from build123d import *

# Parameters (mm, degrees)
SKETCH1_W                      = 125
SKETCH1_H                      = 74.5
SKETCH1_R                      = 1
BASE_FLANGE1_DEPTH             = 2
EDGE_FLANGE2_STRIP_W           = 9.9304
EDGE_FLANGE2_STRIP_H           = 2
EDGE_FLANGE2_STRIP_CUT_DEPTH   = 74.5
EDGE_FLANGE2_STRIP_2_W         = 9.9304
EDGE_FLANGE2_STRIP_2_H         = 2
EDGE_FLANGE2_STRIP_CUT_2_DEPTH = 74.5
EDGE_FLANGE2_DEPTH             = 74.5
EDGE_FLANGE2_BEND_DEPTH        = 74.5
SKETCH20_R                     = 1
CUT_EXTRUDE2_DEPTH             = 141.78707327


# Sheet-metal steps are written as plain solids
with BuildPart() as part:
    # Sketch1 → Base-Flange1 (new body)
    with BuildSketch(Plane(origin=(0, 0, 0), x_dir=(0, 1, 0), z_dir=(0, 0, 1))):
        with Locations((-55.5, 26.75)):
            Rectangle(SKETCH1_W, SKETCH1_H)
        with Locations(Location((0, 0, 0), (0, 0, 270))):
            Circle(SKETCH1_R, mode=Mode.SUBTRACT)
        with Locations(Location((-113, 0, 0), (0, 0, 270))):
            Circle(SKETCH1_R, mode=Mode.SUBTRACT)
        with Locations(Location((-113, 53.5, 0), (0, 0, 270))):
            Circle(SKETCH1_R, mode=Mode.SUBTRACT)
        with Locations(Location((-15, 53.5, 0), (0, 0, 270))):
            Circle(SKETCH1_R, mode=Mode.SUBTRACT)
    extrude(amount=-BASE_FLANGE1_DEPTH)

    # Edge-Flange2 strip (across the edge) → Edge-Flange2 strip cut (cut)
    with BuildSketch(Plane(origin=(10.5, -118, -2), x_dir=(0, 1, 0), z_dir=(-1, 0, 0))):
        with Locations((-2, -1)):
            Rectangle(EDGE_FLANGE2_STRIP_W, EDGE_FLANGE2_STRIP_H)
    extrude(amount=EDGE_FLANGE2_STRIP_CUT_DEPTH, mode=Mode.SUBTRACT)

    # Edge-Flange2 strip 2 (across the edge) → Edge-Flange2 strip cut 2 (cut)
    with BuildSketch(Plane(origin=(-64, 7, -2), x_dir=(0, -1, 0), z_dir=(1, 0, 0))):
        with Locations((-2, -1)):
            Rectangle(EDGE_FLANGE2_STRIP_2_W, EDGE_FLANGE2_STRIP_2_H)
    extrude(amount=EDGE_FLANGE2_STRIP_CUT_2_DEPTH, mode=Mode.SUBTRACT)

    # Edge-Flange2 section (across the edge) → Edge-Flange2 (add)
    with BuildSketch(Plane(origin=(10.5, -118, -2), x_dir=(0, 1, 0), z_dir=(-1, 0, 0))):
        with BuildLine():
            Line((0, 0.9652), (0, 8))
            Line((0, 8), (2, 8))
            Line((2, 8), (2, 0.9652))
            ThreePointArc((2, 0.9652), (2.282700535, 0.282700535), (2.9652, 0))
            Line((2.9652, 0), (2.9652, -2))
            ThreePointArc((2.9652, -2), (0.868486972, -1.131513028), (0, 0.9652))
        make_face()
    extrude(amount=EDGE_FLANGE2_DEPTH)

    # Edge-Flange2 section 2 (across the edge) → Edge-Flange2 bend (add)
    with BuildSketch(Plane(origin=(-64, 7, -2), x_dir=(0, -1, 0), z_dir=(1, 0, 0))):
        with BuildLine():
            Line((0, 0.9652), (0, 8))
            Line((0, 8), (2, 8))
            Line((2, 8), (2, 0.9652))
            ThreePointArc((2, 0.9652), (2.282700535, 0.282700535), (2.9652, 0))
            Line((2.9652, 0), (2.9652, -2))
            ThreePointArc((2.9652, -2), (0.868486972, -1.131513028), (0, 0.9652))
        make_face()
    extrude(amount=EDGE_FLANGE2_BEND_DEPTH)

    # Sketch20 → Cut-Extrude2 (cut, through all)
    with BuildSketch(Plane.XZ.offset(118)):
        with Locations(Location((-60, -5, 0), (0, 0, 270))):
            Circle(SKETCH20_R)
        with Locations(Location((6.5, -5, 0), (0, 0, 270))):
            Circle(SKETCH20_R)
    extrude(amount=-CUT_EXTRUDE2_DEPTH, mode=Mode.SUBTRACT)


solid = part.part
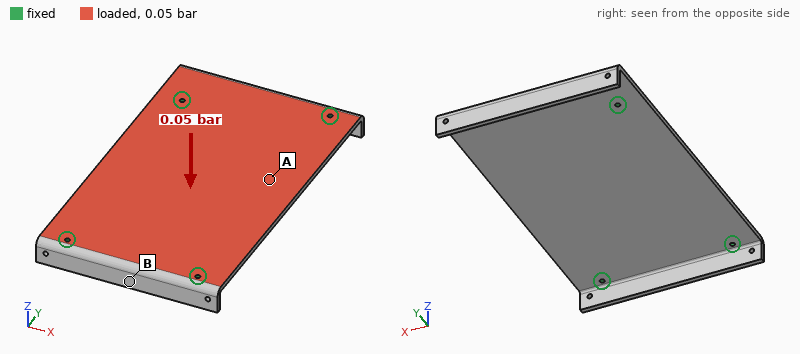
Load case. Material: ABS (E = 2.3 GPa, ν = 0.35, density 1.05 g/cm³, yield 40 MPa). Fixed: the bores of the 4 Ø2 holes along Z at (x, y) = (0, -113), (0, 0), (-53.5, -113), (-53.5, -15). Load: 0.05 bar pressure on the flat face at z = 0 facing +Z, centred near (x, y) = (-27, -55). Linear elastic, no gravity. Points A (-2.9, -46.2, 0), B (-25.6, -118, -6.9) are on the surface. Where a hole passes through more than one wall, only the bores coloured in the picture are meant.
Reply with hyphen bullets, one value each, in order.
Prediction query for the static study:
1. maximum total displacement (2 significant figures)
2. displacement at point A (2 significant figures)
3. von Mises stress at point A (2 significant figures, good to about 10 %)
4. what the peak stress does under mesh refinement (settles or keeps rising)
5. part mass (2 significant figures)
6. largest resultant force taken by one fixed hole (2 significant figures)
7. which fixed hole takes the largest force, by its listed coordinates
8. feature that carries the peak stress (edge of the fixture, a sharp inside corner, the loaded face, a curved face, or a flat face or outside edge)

- 1.7 mm
- 1.5 mm
- 3.4 MPa
- keeps rising
- 22 g
- 15 N
- (-53.5, -15)
- edge of the fixture
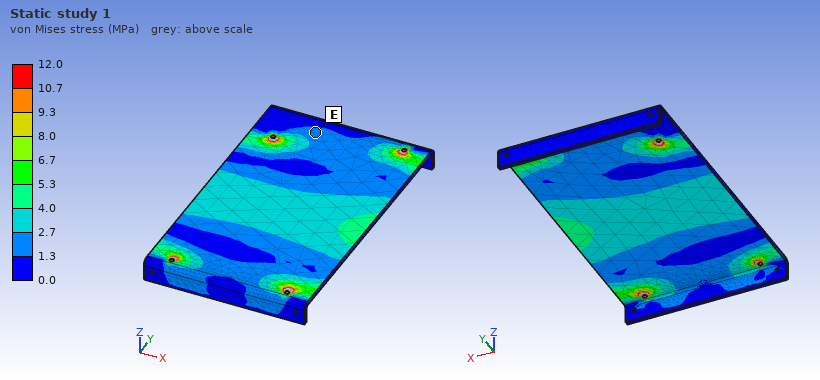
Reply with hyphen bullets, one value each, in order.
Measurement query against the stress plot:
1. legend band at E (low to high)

- 1.3 to 2.7 MPa
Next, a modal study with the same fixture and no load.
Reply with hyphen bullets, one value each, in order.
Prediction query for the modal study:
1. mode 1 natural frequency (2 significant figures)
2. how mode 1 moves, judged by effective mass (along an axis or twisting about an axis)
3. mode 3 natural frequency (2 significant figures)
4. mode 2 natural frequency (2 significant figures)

- 230 Hz
- along Z
- 620 Hz
- 370 Hz
